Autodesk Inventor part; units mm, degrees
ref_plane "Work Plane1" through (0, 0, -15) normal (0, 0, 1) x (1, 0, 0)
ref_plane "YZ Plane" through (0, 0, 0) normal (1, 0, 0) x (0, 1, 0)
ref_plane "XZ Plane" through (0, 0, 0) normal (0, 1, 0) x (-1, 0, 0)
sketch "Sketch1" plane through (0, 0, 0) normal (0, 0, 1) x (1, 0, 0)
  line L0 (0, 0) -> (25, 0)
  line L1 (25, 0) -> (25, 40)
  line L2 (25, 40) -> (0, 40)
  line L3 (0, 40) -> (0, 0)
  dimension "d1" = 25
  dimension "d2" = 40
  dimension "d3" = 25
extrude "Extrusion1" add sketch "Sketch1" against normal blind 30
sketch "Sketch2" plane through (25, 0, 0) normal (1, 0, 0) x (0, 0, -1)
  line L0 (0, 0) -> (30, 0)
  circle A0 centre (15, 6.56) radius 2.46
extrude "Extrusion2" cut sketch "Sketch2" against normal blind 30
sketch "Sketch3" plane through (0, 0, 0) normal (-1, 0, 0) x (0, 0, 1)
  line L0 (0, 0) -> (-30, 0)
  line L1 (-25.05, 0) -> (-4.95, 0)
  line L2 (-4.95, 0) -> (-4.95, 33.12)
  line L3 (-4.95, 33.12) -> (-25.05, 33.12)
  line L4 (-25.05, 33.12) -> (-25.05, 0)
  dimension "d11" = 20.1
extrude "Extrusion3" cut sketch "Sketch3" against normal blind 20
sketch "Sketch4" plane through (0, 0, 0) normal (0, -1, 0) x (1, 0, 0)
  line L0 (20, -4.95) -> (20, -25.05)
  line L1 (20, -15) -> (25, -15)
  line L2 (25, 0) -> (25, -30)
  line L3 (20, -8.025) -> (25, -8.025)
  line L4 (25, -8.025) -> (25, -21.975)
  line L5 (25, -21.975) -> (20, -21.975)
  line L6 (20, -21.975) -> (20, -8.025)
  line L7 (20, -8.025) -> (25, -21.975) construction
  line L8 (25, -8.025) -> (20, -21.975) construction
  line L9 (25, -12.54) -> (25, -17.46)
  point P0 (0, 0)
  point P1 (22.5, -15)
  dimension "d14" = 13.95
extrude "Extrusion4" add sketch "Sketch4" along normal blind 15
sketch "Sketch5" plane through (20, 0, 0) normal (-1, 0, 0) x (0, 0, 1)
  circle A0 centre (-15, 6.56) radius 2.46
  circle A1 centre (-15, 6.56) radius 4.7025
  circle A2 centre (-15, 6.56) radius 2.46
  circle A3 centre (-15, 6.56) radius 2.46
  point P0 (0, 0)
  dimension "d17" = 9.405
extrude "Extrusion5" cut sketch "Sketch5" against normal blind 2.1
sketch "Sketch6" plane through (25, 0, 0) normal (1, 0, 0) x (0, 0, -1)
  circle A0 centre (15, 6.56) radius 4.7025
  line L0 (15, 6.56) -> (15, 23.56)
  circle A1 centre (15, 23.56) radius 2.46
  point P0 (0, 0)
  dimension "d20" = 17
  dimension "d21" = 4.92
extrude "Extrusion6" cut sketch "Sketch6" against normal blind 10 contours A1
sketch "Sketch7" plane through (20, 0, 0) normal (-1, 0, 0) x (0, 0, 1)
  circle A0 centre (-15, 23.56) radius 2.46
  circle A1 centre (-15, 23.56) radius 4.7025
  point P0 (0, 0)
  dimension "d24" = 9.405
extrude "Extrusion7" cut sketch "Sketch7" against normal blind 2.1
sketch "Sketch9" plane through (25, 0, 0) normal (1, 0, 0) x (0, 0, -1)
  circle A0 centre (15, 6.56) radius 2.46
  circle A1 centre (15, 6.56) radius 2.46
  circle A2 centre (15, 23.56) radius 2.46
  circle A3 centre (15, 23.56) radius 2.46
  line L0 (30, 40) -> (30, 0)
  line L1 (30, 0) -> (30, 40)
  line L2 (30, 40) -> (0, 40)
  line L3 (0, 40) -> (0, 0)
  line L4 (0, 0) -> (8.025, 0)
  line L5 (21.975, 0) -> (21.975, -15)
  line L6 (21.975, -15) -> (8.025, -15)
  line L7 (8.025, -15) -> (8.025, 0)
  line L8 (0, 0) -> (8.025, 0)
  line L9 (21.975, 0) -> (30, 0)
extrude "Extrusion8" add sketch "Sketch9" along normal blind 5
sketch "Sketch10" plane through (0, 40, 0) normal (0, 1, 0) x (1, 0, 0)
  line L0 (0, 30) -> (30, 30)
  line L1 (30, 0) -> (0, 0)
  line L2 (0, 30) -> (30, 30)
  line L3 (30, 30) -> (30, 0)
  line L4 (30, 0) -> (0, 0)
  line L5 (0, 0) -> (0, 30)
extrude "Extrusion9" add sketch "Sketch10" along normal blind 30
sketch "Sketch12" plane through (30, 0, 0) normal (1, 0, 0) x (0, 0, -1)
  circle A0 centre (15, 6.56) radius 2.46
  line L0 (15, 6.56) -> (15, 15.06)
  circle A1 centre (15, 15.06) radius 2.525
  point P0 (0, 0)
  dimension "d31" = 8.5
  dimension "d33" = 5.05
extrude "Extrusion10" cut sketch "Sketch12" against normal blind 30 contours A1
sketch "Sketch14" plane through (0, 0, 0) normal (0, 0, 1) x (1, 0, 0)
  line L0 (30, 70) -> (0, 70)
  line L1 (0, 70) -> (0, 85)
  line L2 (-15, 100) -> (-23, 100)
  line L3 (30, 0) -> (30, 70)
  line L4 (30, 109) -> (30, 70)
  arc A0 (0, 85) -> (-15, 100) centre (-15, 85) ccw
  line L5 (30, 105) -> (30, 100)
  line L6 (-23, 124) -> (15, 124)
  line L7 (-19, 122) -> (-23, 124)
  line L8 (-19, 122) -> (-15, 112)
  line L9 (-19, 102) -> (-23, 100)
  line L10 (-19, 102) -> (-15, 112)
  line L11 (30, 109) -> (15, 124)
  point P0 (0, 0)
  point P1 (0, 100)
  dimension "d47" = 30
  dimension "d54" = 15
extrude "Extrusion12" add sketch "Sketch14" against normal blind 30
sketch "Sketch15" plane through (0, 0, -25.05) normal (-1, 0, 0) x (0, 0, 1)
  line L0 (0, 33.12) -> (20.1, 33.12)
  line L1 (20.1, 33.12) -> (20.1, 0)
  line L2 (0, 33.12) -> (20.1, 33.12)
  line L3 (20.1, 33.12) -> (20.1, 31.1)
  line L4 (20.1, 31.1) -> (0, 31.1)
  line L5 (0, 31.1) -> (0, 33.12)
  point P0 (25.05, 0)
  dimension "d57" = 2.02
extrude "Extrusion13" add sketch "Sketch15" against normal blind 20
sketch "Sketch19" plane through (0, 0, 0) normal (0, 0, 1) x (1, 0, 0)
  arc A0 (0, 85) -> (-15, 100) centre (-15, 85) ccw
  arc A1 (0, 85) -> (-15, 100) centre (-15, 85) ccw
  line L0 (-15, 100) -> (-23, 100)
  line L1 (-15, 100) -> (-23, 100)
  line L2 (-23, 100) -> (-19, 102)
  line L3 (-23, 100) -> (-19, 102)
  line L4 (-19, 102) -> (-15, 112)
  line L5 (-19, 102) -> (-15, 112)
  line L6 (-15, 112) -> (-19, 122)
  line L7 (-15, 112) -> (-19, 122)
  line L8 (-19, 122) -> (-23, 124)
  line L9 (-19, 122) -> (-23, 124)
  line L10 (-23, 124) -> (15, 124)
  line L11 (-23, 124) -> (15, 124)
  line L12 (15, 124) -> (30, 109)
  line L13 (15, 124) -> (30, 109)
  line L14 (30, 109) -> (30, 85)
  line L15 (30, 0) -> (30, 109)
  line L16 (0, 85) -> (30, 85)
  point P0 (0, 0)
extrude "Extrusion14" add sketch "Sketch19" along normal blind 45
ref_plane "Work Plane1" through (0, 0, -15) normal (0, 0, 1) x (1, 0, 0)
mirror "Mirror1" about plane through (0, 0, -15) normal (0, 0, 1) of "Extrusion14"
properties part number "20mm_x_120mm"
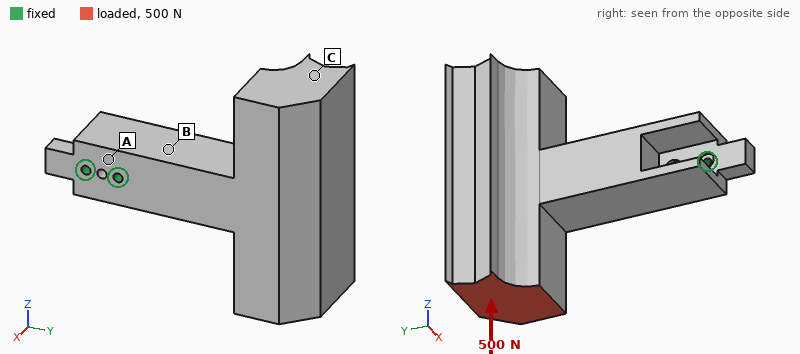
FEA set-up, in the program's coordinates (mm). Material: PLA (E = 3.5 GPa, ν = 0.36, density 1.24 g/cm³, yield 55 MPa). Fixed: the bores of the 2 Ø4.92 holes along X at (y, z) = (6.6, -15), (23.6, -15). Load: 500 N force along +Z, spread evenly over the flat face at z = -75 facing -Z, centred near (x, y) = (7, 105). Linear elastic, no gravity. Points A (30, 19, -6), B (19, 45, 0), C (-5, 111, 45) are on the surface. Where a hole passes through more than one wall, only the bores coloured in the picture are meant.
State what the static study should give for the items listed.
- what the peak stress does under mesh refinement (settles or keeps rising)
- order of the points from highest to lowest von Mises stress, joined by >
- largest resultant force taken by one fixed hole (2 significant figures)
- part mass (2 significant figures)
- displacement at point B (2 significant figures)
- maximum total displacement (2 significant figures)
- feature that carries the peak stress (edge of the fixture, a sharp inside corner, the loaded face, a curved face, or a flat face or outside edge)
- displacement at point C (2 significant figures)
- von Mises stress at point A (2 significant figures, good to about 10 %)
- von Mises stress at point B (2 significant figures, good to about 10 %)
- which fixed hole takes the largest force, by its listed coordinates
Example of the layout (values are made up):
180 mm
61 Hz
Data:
keeps rising
A > B > C
2.3 kN
310 g
0.38 mm
2.2 mm
edge of the fixture
1.9 mm
15 MPa
7.6 MPa
(23.6, -15)
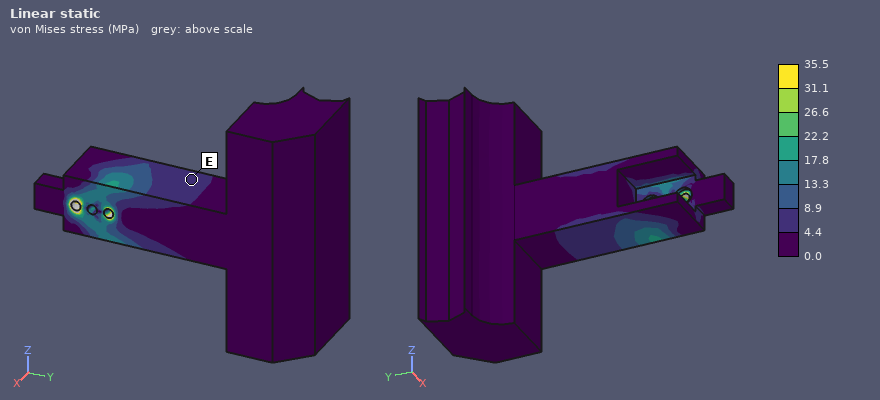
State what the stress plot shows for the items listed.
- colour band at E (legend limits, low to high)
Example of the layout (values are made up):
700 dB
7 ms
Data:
4.4 to 8.9 MPa
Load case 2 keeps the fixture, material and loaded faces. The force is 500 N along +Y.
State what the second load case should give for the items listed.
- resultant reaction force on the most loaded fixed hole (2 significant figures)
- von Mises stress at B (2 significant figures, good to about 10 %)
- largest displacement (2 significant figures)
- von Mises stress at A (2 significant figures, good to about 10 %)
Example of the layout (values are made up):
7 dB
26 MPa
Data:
1.4 kN
7.4 MPa
2.0 mm
12 MPa
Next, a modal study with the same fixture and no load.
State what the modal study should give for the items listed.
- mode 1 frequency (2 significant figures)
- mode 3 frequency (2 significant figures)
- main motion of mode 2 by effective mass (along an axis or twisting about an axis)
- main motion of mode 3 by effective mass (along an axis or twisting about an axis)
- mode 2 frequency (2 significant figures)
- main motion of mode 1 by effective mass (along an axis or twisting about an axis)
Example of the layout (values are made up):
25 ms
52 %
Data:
160 Hz
250 Hz
along Z
twisting about Y
180 Hz
along X
